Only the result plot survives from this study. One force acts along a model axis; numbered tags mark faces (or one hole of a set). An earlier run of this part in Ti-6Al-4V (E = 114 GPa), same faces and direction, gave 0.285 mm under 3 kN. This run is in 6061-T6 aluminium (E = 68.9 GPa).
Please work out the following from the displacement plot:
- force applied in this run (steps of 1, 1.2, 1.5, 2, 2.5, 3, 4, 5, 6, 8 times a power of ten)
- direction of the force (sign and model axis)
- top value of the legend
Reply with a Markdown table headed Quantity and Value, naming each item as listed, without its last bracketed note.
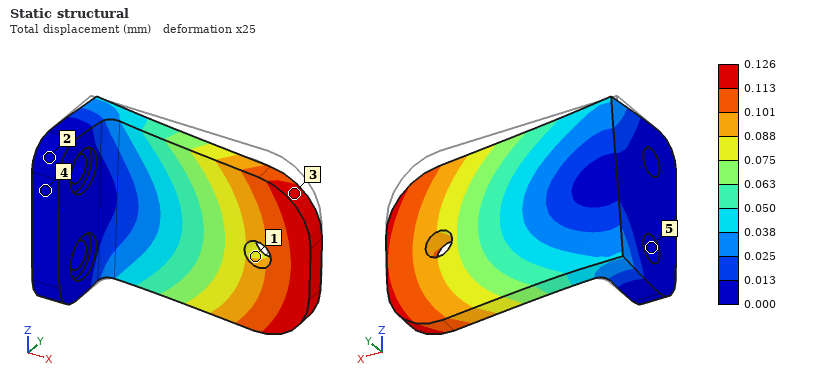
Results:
| Quantity | Value |
|---|---|
| force applied in this run | 800 N |
| direction of the force | -Z |
| top value of the legend | 0.126 mm |
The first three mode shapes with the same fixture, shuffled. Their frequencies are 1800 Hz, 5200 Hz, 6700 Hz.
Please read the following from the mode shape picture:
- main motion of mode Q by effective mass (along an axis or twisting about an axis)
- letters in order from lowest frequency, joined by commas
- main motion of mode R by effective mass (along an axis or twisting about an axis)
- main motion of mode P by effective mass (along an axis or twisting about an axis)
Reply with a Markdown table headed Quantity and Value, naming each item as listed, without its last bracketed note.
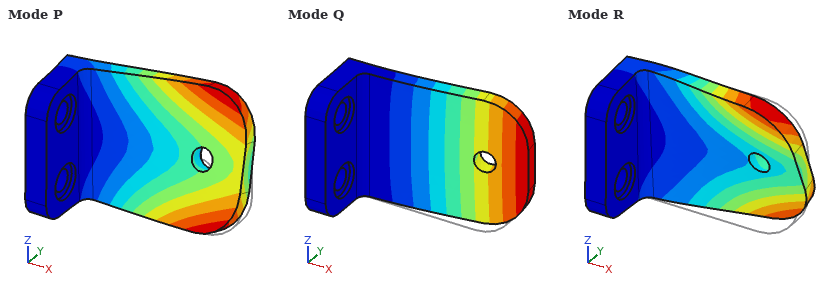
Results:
| Quantity | Value |
|---|---|
| main motion of mode Q by effective mass | along Y |
| letters in order from lowest frequency, joined by commas | Q, P, R |
| main motion of mode R by effective mass | along Z |
| main motion of mode P by effective mass | along Z |
